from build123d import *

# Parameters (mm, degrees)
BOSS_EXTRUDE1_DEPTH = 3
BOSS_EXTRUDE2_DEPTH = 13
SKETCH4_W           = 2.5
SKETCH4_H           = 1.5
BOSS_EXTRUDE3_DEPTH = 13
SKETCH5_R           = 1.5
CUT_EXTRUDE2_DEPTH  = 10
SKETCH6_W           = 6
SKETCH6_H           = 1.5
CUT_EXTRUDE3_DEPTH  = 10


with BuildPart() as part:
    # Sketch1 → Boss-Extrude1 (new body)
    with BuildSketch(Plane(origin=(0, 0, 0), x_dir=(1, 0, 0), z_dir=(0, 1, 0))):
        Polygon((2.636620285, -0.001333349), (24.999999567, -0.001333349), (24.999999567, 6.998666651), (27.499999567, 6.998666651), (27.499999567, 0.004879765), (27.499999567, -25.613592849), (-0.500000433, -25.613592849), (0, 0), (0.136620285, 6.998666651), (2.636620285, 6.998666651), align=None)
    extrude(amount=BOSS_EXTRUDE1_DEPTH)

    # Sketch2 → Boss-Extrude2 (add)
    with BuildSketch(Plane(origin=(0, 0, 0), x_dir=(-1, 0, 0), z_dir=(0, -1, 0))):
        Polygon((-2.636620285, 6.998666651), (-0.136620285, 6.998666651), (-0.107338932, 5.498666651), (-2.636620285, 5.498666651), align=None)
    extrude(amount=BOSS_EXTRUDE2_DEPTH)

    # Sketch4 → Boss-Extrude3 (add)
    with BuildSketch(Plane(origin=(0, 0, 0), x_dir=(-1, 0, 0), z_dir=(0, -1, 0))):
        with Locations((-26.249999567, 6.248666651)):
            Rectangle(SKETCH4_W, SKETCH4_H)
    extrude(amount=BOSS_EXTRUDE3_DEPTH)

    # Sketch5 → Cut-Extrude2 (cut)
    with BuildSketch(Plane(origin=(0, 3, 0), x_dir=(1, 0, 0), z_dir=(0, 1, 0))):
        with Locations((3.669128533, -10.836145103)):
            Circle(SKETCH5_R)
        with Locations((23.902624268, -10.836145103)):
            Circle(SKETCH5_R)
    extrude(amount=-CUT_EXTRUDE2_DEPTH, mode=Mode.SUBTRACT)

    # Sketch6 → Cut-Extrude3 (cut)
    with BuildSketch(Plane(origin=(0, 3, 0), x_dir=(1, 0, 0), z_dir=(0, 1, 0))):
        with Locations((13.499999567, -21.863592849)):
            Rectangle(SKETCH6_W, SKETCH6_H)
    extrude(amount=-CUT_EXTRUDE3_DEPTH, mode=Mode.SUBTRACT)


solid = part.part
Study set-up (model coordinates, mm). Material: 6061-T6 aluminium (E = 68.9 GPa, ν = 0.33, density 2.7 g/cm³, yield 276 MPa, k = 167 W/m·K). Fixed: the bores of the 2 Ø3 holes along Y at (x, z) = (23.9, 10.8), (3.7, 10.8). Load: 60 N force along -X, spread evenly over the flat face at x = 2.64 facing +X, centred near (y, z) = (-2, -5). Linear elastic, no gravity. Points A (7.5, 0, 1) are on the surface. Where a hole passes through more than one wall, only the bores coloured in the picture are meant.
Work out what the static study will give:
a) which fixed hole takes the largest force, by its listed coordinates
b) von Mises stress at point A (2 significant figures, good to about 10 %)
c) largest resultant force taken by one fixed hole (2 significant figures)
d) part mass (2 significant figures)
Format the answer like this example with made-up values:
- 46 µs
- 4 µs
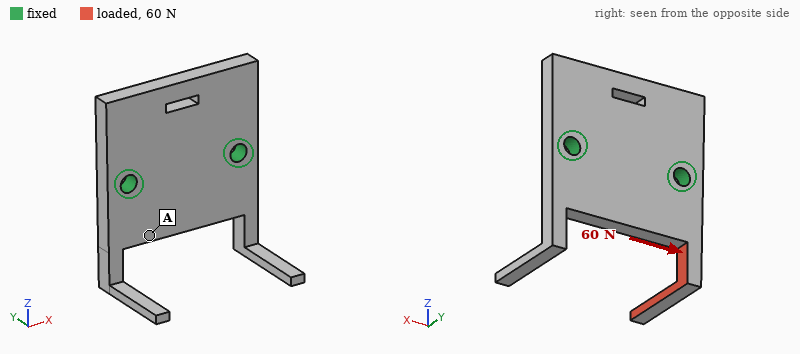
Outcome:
- (23.9, 10.8)
- 17 MPa
- 59 N
- 6.1 g
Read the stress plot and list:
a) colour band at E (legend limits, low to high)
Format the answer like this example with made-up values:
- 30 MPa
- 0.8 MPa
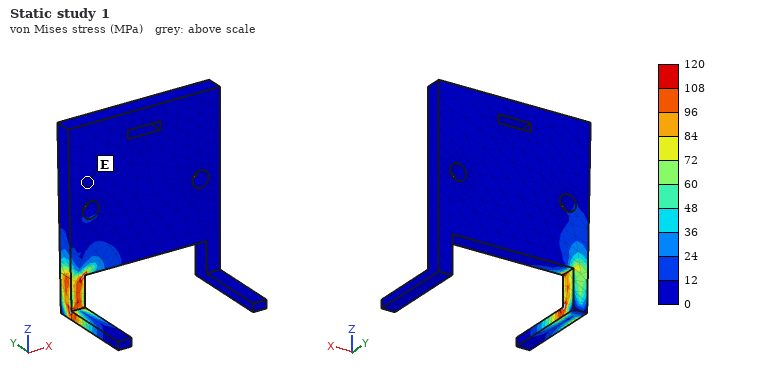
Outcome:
- 0 to 12 MPa
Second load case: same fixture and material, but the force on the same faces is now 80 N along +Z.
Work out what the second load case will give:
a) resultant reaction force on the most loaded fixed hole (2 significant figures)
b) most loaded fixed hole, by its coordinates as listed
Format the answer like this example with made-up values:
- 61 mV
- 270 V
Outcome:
- 82 N
- (3.7, 10.8)
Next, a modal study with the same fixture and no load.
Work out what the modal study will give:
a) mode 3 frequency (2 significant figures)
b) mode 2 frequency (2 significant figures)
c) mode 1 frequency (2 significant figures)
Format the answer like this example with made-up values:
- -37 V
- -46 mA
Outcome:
- 6000 Hz
- 5200 Hz
- 5200 Hz
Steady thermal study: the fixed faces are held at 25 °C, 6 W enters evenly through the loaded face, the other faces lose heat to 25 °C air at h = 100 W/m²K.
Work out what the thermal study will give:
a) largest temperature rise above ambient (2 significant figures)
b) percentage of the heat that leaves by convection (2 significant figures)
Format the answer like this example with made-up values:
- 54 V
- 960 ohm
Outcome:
- 63 K
- 15 %
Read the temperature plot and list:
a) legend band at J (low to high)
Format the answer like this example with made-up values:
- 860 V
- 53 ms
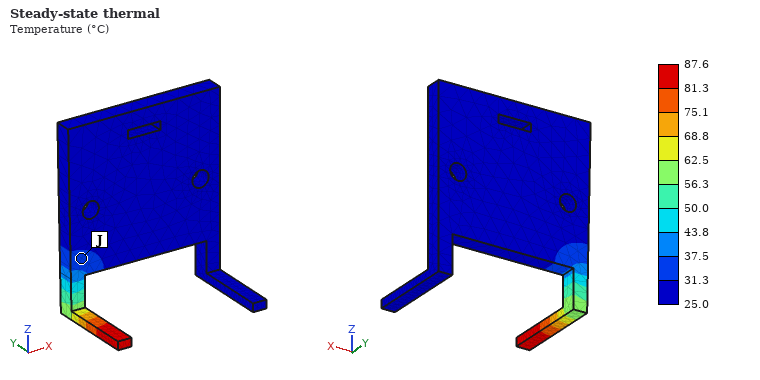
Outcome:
- 31.3 to 37.5 °C
